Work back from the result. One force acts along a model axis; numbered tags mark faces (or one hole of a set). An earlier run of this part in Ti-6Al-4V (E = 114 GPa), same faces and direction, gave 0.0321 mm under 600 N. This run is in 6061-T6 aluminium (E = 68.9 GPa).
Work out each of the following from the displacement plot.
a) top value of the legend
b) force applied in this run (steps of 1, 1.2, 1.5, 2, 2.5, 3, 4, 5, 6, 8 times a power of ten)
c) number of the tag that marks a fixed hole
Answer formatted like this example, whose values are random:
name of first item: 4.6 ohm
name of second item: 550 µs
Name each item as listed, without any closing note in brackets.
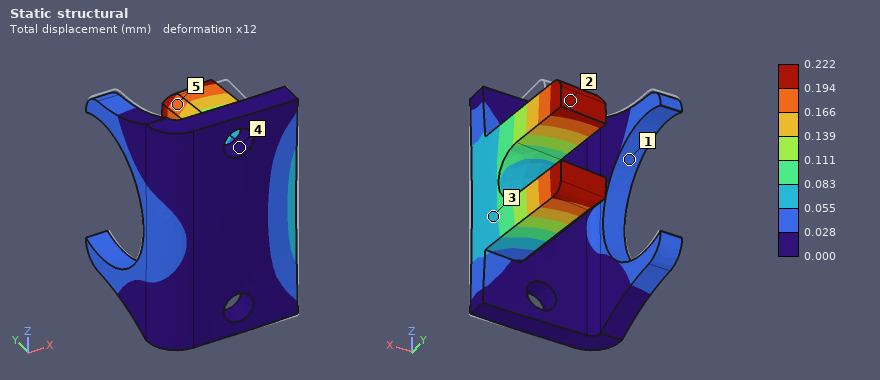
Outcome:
top value of the legend: 0.222 mm
force applied in this run: 2.5 kN
number of the tag that marks a fixed hole: 4
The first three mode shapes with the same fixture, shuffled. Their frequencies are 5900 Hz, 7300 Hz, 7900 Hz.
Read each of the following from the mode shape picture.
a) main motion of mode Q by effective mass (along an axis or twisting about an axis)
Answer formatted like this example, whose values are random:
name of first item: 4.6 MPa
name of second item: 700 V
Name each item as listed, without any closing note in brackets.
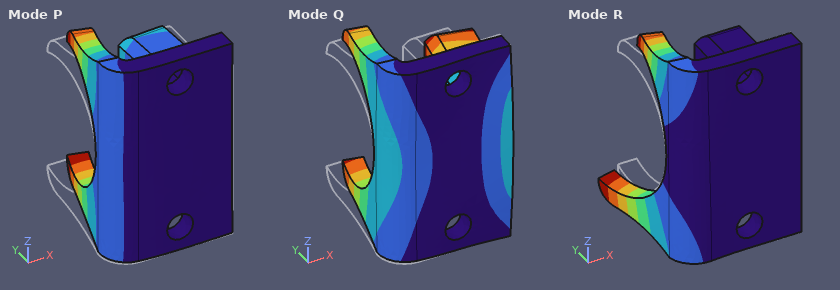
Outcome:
main motion of mode Q by effective mass: along X
